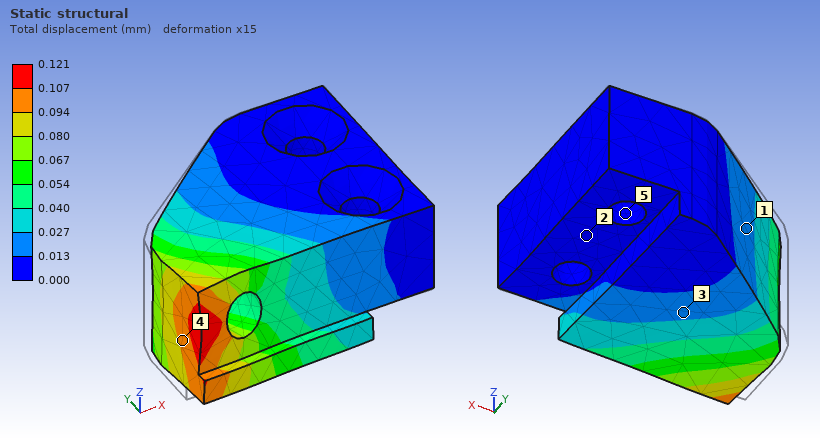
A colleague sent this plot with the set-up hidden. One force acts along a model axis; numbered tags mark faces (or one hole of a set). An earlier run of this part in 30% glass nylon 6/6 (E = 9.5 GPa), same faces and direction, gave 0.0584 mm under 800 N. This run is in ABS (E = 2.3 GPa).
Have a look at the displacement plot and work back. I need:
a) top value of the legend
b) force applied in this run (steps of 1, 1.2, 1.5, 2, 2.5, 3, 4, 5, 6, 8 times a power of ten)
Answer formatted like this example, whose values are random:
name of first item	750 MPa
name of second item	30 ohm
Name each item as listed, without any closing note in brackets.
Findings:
top value of the legend	0.121 mm
force applied in this run	400 N
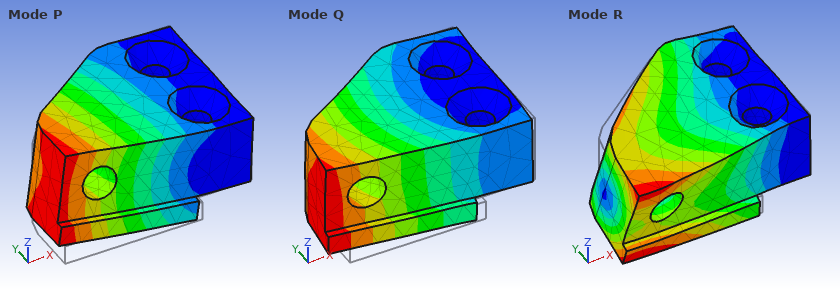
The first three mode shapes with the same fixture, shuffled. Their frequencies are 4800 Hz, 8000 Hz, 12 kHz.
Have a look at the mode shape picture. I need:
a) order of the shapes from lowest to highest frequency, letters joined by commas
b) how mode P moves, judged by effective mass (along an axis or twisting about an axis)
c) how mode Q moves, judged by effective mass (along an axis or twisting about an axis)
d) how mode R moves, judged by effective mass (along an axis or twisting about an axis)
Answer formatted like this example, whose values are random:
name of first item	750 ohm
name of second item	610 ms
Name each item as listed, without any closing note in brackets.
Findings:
order of the shapes from lowest to highest frequency, letters joined by commas	P, Q, R
how mode P moves, judged by effective mass	along Z
how mode Q moves, judged by effective mass	along Y
how mode R moves, judged by effective mass	twisting about X
